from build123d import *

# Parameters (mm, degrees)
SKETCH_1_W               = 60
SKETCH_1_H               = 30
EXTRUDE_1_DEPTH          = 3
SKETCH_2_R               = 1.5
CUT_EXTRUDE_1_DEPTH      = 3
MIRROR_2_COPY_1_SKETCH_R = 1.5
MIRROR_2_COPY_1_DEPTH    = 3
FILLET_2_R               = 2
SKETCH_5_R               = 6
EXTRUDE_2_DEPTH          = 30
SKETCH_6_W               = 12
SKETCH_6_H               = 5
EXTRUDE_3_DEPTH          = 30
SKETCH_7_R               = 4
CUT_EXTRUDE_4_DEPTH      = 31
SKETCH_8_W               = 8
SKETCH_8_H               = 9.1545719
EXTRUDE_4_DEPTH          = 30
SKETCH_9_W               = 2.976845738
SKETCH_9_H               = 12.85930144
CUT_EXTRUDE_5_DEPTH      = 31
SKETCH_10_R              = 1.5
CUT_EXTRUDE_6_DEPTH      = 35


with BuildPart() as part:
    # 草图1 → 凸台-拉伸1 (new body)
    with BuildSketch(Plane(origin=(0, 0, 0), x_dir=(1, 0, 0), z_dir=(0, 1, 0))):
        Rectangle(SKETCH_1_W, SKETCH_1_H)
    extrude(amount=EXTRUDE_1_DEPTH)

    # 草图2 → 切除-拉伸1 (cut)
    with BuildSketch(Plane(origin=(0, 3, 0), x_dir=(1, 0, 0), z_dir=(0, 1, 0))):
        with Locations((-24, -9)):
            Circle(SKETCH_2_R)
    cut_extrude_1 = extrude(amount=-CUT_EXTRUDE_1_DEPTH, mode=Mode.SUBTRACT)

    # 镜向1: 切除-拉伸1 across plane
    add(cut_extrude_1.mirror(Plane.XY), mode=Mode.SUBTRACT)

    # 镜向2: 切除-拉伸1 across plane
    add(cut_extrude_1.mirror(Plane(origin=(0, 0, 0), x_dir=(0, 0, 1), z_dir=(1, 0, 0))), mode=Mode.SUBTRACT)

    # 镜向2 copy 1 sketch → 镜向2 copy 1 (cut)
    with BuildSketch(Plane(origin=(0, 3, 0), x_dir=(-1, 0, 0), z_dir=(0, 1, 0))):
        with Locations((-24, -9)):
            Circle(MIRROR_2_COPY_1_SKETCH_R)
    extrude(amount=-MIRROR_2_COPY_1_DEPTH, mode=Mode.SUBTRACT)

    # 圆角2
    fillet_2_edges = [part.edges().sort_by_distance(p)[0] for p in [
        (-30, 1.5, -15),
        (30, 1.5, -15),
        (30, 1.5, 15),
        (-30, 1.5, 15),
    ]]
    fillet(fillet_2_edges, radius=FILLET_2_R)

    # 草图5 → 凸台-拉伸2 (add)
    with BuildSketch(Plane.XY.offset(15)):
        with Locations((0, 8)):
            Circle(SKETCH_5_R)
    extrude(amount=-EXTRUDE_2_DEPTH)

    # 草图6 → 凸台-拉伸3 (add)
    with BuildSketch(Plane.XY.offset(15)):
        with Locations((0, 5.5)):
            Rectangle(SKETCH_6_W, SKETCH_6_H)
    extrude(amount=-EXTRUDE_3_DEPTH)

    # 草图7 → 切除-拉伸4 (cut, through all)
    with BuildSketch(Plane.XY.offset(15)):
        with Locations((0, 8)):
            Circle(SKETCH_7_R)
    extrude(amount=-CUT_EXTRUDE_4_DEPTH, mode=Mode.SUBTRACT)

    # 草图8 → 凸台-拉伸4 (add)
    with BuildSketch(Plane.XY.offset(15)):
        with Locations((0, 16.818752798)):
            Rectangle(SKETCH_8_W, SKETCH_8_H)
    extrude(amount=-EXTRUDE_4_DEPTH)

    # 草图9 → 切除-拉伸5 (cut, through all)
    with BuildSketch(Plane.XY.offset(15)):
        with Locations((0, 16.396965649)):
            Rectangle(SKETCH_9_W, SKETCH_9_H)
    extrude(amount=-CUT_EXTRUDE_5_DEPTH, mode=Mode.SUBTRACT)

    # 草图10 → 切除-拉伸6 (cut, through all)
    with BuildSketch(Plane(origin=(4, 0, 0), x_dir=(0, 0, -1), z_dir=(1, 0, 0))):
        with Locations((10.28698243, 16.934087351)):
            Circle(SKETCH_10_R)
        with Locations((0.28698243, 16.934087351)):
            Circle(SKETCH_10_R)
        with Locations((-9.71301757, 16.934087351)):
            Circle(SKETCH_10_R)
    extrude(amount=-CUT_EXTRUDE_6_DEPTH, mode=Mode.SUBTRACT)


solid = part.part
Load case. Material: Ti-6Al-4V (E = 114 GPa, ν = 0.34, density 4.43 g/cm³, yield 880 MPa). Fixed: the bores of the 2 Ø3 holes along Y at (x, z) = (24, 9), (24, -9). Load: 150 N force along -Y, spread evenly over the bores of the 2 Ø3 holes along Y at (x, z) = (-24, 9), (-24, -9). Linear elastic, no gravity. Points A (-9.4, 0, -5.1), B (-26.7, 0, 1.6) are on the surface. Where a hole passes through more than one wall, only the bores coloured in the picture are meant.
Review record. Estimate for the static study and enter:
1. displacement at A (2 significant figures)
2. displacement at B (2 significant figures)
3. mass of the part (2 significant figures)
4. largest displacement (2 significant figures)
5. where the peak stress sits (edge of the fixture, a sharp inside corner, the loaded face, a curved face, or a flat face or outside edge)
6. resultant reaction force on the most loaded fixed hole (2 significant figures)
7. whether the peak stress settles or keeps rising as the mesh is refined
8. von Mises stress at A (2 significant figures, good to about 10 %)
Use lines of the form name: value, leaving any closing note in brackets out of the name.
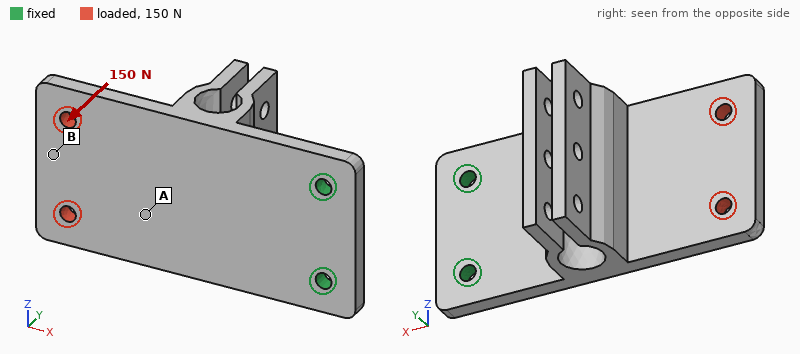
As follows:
displacement at A: 0.36 mm
displacement at B: 0.66 mm
mass of the part: 36 g
largest displacement: 0.72 mm
where the peak stress sits: edge of the fixture
resultant reaction force on the most loaded fixed hole: 75 N
whether the peak stress settles or keeps rising as the mesh is refined: keeps rising
von Mises stress at A: 43 MPa
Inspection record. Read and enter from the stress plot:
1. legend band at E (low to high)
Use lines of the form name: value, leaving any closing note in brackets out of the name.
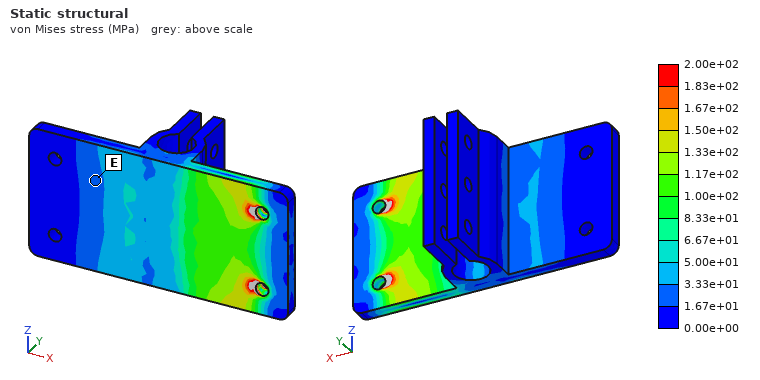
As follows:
legend band at E: 1.67e+01 to 3.33e+01 MPa
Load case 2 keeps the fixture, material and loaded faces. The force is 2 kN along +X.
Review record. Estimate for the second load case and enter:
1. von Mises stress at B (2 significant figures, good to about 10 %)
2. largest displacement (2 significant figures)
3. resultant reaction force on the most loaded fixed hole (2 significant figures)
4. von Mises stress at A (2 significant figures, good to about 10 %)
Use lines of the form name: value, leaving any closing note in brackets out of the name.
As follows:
von Mises stress at B: 8.0 MPa
largest displacement: 21 µm
resultant reaction force on the most loaded fixed hole: 1.0 kN
von Mises stress at A: 22 MPa
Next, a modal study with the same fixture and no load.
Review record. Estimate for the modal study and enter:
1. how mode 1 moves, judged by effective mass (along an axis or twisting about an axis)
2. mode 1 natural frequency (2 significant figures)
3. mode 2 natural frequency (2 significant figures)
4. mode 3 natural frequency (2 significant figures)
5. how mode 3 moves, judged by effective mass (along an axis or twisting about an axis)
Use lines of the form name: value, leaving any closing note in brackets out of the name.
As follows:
how mode 1 moves, judged by effective mass: along Y
mode 1 natural frequency: 780 Hz
mode 2 natural frequency: 2600 Hz
mode 3 natural frequency: 4400 Hz
how mode 3 moves, judged by effective mass: along Y
